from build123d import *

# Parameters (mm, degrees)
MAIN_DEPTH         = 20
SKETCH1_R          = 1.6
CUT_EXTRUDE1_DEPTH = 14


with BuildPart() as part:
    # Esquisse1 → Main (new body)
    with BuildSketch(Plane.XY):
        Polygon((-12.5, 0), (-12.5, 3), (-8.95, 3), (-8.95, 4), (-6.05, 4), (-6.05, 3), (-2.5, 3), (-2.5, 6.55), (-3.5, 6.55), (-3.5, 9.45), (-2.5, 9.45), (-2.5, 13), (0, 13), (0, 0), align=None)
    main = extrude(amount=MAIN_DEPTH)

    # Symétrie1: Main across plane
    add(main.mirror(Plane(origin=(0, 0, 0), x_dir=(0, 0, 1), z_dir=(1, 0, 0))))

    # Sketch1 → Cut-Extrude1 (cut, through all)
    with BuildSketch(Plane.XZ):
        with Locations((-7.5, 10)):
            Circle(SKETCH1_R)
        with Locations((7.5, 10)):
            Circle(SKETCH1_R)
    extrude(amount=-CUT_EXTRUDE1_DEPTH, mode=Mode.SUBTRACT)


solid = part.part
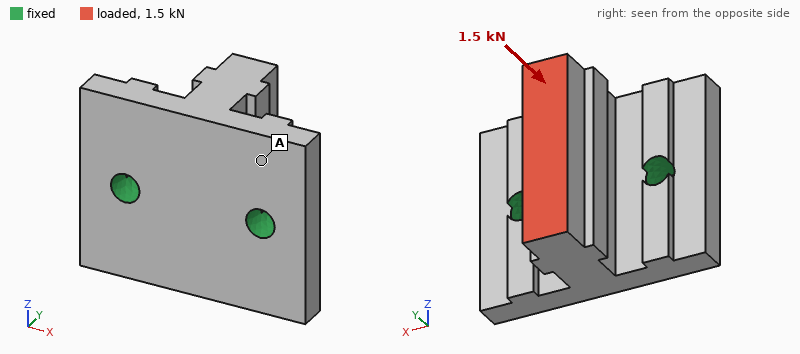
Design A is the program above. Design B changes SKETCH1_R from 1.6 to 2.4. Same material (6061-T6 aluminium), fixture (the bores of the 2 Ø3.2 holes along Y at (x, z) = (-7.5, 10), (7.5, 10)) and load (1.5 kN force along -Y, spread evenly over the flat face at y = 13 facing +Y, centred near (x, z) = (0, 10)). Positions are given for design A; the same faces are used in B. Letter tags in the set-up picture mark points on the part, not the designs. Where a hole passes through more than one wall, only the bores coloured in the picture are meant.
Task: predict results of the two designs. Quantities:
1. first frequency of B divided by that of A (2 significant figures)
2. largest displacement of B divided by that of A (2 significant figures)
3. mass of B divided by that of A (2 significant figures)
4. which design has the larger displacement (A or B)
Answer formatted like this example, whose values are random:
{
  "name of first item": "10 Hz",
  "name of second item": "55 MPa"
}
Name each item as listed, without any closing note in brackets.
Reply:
{
  "first frequency of B divided by that of A": "1.2",
  "largest displacement of B divided by that of A": "0.75",
  "mass of B divided by that of A": "0.97",
  "which design has the larger displacement": "A"
}
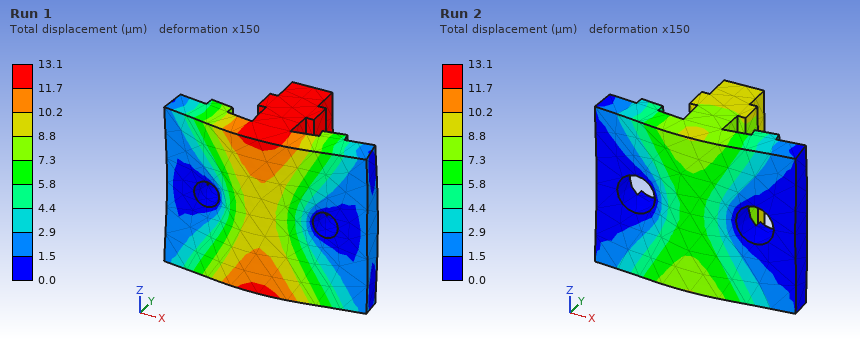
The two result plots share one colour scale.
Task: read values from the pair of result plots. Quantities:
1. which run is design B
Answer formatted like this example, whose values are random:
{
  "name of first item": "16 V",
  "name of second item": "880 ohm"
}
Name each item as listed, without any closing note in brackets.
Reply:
{
  "which run is design B": "Run 2"
}
